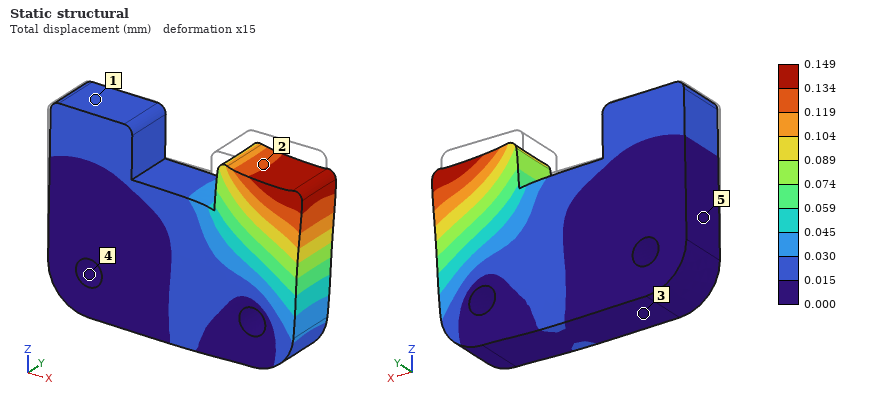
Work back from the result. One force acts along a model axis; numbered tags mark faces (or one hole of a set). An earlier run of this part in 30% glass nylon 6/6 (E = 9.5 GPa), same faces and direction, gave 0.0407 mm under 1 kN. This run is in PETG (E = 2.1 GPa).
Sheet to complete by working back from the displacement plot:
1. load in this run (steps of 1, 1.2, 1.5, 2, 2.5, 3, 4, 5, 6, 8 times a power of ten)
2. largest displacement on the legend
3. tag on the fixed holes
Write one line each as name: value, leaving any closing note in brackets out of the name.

load in this run: 800 N
largest displacement on the legend: 0.149 mm
tag on the fixed holes: 4
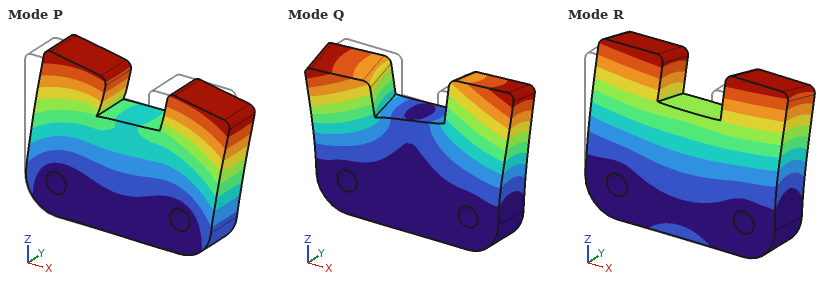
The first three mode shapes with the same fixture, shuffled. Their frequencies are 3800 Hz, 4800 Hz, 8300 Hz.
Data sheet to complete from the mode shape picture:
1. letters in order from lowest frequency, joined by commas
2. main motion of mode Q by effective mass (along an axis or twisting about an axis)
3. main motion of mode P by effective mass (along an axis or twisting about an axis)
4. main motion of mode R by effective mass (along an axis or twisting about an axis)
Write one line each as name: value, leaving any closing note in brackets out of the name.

letters in order from lowest frequency, joined by commas: R, Q, P
main motion of mode Q by effective mass: twisting about Z
main motion of mode P by effective mass: along X
main motion of mode R by effective mass: along Y
